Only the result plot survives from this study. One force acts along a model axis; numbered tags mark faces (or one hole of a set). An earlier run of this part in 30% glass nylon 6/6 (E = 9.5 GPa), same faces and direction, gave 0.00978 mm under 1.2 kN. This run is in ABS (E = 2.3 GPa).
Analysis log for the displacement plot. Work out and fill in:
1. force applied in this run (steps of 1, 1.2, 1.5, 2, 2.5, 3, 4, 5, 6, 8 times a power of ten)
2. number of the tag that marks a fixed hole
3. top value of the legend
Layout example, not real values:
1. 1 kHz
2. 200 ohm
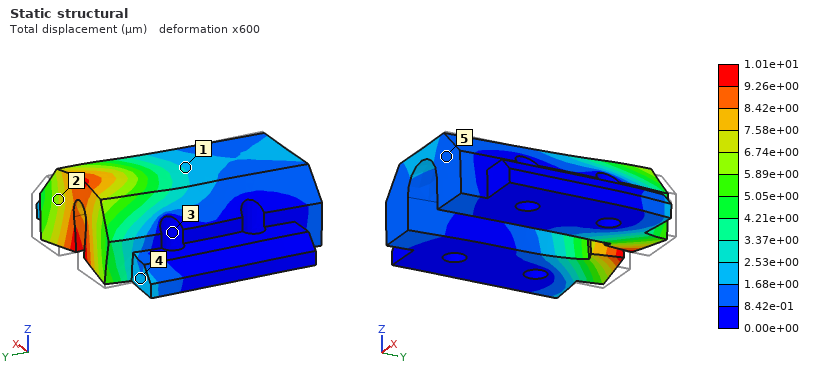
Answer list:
1. 300 N
2. 3
3. 1.01e+01 µm
